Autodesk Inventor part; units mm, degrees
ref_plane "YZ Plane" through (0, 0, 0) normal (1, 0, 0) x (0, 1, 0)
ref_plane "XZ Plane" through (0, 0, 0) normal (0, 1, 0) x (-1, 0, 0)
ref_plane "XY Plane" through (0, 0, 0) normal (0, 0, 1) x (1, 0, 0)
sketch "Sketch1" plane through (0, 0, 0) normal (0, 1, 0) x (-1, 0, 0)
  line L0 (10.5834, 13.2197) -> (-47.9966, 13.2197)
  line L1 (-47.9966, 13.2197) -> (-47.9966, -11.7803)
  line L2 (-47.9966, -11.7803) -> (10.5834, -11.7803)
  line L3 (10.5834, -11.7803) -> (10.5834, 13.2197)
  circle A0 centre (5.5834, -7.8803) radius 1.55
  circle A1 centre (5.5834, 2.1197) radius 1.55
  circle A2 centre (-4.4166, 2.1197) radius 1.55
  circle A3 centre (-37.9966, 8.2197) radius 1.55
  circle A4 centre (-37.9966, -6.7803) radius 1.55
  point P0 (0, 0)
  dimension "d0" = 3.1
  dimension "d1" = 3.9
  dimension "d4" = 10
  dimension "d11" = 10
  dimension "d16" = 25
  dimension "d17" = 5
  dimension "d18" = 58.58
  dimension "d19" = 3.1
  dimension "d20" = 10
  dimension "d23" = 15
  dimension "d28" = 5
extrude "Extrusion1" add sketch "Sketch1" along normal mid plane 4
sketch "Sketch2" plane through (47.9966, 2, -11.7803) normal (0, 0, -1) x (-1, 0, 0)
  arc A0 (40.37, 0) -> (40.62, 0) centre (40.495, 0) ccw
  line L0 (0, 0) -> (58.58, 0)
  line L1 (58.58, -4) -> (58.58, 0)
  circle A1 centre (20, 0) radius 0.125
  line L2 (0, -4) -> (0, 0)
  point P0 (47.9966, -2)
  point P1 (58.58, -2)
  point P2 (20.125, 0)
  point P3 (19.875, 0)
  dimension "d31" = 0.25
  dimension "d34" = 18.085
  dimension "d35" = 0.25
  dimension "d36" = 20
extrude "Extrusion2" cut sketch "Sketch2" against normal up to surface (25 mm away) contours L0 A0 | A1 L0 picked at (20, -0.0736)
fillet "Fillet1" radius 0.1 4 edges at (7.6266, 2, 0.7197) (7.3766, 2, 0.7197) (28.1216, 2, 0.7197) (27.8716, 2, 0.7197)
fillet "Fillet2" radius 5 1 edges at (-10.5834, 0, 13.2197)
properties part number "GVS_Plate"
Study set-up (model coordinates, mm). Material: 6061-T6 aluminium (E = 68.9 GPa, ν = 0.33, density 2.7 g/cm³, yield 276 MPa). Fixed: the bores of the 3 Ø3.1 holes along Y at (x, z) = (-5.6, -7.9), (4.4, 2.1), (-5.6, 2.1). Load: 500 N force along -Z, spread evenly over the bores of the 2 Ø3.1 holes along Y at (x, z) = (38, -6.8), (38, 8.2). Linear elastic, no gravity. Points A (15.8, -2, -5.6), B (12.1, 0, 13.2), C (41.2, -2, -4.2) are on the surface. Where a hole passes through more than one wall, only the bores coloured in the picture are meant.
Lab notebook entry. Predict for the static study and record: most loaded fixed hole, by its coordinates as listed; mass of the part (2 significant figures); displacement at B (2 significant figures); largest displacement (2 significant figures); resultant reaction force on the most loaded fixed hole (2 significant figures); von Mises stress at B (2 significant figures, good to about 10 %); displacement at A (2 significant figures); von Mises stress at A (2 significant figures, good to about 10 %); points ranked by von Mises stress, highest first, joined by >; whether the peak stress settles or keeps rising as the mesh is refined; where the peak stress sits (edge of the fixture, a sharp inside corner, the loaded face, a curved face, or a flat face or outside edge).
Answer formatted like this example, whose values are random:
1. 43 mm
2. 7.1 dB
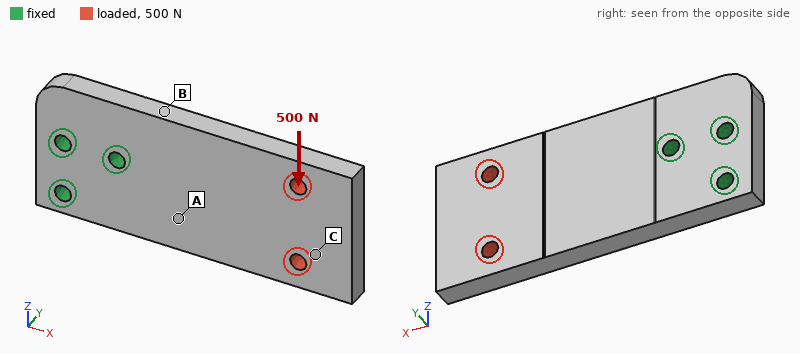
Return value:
1. (4.4, 2.1)
2. 15 g
3. 14 µm
4. 59 µm
5. 1.2 kN
6. 30 MPa
7. 13 µm
8. 17 MPa
9. B > A > C
10. keeps rising
11. edge of the fixture
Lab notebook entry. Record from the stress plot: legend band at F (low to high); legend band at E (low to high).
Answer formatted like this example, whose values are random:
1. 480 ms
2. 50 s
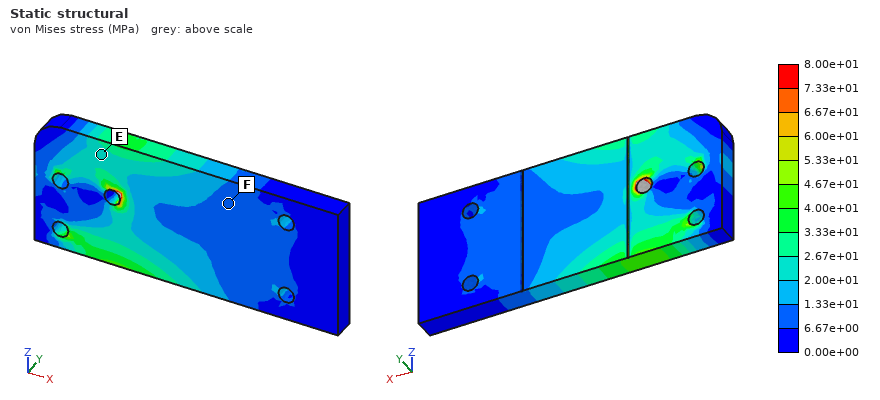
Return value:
1. 6.67e+00 to 1.33e+01 MPa
2. 2.00e+01 to 2.67e+01 MPa
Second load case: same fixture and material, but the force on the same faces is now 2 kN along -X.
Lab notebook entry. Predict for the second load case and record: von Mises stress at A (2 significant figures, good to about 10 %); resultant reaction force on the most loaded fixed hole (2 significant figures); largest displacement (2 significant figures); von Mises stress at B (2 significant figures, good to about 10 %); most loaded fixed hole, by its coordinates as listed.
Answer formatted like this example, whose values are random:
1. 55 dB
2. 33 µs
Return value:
1. 20 MPa
2. 1.2 kN
3. 13 µm
4. 14 MPa
5. (4.4, 2.1)
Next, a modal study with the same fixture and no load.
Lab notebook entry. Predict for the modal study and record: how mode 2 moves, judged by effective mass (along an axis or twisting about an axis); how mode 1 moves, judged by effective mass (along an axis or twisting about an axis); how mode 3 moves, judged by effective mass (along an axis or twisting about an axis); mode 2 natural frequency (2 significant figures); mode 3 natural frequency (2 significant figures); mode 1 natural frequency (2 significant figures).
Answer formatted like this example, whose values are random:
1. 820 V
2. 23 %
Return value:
1. twisting about X
2. along Y
3. along Z
4. 5400 Hz
5. 6700 Hz
6. 1700 Hz
